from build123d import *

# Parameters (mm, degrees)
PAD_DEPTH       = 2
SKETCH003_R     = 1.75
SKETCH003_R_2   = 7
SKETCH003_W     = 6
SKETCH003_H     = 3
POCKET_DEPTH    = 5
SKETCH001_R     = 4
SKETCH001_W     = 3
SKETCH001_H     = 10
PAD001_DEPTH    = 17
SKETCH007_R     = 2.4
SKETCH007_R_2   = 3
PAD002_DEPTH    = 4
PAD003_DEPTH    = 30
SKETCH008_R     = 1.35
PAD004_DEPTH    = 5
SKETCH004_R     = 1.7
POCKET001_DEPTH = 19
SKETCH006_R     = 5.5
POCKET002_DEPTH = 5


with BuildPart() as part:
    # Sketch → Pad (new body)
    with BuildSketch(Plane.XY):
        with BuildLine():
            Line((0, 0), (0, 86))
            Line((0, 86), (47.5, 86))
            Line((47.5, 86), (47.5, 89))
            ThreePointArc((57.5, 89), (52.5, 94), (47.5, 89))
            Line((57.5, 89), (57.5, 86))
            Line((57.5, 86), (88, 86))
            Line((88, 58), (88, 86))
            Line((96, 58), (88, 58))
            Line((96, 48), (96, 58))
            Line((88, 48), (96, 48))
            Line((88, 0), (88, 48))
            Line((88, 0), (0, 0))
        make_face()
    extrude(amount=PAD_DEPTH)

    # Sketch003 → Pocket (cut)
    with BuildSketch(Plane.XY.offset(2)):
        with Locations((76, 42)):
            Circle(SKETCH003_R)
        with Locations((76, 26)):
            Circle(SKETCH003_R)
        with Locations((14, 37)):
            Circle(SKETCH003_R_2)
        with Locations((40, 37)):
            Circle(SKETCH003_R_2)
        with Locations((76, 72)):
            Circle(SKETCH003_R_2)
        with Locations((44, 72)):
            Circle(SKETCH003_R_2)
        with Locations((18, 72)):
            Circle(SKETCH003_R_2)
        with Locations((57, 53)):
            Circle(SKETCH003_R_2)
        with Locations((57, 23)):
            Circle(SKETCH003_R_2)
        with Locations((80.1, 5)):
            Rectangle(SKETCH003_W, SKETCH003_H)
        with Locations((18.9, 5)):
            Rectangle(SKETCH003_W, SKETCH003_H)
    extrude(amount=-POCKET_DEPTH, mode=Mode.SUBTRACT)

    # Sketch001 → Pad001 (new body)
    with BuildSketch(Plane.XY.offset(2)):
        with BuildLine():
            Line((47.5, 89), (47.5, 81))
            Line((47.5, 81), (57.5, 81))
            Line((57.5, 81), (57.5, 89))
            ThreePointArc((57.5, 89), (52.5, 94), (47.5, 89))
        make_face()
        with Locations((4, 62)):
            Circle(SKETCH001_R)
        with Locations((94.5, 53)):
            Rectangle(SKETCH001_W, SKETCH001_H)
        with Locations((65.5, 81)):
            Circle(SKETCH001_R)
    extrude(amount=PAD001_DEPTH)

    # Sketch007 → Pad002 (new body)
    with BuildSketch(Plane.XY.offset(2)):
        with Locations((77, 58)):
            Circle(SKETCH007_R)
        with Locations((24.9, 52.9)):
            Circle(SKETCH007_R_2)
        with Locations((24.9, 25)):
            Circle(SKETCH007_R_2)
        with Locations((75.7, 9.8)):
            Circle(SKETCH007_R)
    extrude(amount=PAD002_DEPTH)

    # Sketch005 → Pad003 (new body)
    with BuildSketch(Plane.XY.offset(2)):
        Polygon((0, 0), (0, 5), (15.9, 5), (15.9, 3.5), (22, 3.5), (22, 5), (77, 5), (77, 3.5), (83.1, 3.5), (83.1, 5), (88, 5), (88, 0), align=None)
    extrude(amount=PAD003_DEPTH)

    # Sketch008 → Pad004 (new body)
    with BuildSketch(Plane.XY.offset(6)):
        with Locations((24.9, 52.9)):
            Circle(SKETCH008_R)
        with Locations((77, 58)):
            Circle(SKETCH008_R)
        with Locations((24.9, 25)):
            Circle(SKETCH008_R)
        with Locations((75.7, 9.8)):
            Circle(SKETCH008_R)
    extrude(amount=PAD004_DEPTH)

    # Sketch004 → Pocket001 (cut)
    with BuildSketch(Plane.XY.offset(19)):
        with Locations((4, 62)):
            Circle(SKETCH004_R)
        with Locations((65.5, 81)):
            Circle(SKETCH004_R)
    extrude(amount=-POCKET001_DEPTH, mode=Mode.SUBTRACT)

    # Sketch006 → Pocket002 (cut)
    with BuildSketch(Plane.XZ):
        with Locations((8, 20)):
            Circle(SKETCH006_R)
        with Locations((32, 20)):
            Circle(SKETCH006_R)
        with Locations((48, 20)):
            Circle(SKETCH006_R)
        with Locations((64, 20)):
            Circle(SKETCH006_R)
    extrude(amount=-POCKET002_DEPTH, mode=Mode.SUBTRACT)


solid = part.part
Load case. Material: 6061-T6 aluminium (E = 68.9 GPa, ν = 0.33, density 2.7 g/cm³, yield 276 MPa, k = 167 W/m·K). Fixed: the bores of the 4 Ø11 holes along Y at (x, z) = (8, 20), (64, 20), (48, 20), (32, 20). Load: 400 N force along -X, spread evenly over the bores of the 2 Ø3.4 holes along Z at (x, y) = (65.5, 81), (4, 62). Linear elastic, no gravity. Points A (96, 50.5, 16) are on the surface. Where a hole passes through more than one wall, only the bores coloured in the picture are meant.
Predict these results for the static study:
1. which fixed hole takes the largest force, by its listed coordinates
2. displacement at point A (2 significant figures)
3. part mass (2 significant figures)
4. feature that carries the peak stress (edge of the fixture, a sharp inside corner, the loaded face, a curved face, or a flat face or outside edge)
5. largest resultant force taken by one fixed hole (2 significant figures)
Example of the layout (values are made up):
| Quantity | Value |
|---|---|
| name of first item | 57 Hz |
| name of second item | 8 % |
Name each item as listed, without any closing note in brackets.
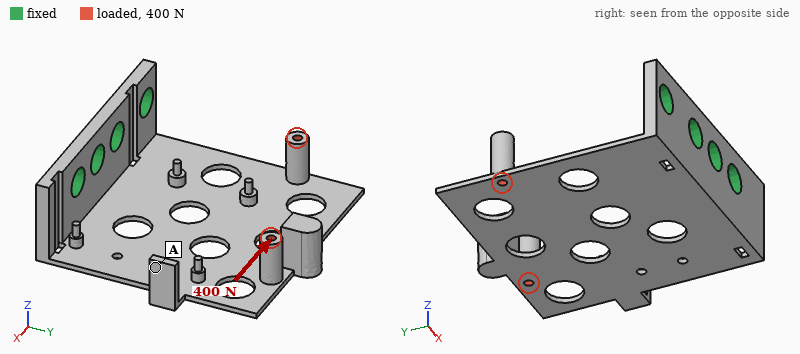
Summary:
| Quantity | Value |
|---|---|
| which fixed hole takes the largest force, by its listed coordinates | (64, 20) |
| displacement at point A | 1.0 mm |
| part mass | 76 g |
| feature that carries the peak stress | a flat face or outside edge |
| largest resultant force taken by one fixed hole | 460 N |
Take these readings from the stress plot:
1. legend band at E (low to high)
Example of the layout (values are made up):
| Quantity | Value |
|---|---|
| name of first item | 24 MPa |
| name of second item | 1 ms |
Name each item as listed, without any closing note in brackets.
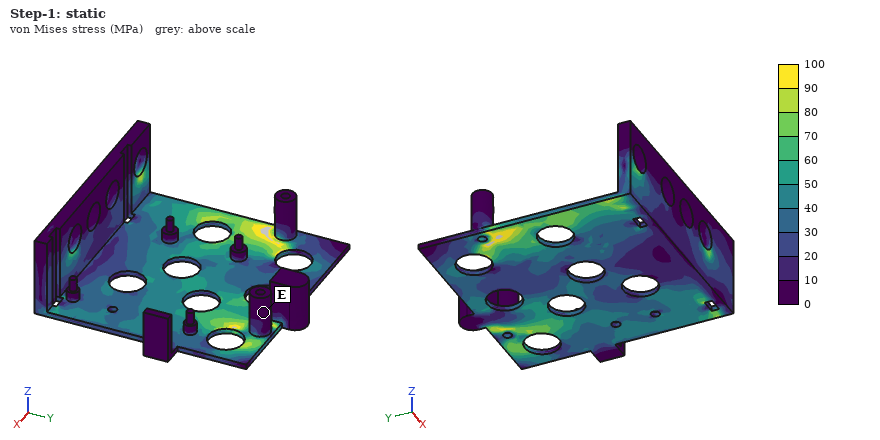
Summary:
| Quantity | Value |
|---|---|
| legend band at E | 0 to 10 MPa |
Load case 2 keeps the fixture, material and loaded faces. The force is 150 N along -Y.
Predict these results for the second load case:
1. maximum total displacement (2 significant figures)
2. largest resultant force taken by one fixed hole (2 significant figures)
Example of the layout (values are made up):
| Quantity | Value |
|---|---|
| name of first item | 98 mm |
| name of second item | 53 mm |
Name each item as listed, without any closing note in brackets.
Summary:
| Quantity | Value |
|---|---|
| maximum total displacement | 1.5 mm |
| largest resultant force taken by one fixed hole | 48 N |
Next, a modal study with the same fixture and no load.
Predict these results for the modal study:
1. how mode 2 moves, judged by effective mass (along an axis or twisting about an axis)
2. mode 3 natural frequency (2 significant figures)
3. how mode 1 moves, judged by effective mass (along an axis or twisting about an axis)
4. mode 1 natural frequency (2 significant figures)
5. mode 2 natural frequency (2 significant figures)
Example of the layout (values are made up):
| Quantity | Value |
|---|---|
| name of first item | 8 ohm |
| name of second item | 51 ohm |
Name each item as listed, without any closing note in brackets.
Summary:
| Quantity | Value |
|---|---|
| how mode 2 moves, judged by effective mass | twisting about Y |
| mode 3 natural frequency | 800 Hz |
| how mode 1 moves, judged by effective mass | along Z |
| mode 1 natural frequency | 170 Hz |
| mode 2 natural frequency | 430 Hz |
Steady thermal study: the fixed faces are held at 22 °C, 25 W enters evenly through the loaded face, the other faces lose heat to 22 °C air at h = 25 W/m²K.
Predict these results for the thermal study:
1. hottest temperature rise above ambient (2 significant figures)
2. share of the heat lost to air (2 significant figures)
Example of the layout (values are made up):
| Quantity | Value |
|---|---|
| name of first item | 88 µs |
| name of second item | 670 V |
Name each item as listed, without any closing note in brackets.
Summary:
| Quantity | Value |
|---|---|
| hottest temperature rise above ambient | 72 K |
| share of the heat lost to air | 50 % |
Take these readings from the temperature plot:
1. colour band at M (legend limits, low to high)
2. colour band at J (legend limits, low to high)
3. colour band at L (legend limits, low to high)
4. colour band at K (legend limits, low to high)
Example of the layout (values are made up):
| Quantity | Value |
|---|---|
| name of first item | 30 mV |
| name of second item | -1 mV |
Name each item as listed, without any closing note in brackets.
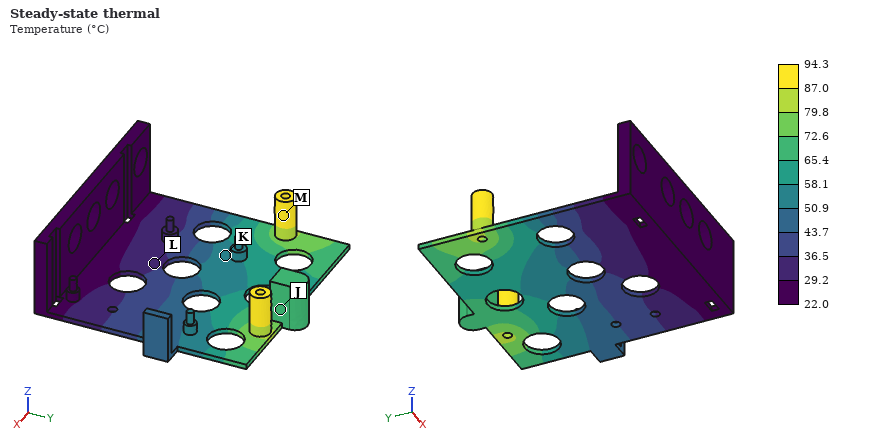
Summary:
| Quantity | Value |
|---|---|
| colour band at M | 87.0 to 94.3 °C |
| colour band at J | 65.4 to 72.6 °C |
| colour band at L | 29.2 to 36.5 °C |
| colour band at K | 50.9 to 58.1 °C |
